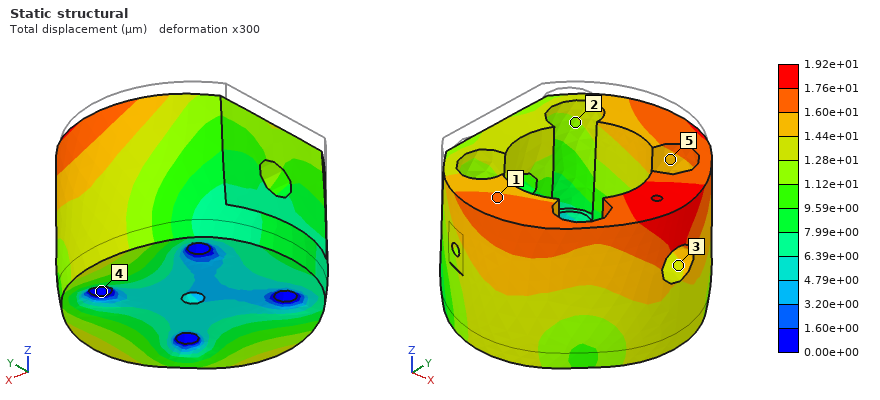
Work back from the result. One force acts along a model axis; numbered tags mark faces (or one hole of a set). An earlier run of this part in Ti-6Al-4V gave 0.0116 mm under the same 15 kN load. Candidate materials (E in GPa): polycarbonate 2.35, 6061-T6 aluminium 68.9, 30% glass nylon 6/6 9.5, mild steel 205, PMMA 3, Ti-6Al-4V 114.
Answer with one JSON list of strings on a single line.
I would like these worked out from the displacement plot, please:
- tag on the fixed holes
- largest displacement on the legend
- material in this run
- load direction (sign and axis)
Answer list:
["4", "1.92e+01 µm", "6061-T6 aluminium", "-Z"]
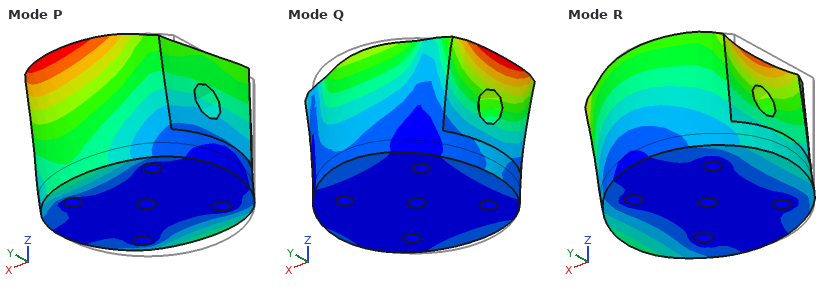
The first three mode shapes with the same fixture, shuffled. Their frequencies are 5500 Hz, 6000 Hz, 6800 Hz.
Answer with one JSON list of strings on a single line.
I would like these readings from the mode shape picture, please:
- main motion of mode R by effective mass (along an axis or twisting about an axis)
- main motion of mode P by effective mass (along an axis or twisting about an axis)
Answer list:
["along X", "along Y"]
